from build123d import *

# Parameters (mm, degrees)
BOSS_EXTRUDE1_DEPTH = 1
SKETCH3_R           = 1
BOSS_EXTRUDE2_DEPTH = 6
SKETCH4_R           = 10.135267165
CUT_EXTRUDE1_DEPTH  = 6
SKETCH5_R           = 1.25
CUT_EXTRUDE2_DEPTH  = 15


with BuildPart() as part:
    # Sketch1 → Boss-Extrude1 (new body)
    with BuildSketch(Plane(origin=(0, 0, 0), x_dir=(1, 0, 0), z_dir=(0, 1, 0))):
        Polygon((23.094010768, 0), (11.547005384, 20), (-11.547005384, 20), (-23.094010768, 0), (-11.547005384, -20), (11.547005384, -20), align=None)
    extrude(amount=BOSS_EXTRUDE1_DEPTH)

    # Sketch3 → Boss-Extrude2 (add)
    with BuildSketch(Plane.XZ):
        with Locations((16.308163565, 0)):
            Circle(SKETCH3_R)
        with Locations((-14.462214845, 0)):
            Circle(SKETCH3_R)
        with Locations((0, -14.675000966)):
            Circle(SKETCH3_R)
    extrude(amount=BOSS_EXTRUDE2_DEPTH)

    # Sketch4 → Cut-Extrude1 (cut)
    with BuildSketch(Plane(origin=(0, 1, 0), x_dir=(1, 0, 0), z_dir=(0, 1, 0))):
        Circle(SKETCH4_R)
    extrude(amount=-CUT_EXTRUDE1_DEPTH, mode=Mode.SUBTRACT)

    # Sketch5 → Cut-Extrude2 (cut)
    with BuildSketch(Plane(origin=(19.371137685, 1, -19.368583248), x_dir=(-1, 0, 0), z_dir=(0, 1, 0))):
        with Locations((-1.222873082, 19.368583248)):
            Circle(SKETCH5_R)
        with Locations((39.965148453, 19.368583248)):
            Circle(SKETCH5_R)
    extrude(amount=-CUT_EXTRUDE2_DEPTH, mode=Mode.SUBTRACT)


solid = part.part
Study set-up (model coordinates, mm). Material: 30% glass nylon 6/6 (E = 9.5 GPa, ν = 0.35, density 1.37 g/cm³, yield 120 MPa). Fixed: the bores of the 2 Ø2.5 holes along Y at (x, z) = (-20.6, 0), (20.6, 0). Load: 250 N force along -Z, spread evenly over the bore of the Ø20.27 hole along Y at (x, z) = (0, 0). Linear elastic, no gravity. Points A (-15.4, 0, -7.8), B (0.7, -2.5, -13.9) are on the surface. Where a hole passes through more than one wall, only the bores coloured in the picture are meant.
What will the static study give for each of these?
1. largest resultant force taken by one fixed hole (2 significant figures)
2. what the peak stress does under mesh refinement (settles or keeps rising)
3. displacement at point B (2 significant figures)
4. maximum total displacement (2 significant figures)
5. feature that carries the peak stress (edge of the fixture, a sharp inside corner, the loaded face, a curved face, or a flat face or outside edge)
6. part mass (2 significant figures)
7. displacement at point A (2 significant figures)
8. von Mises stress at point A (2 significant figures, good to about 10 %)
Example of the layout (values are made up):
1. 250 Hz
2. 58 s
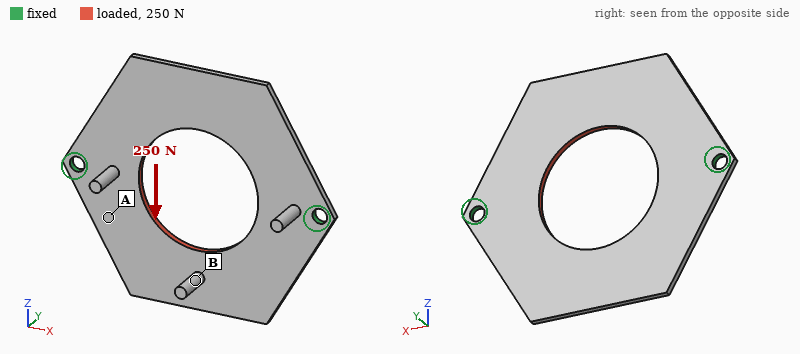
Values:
1. 130 N
2. keeps rising
3. 31 µm
4. 33 µm
5. edge of the fixture
6. 1.5 g
7. 20 µm
8. 9.7 MPa
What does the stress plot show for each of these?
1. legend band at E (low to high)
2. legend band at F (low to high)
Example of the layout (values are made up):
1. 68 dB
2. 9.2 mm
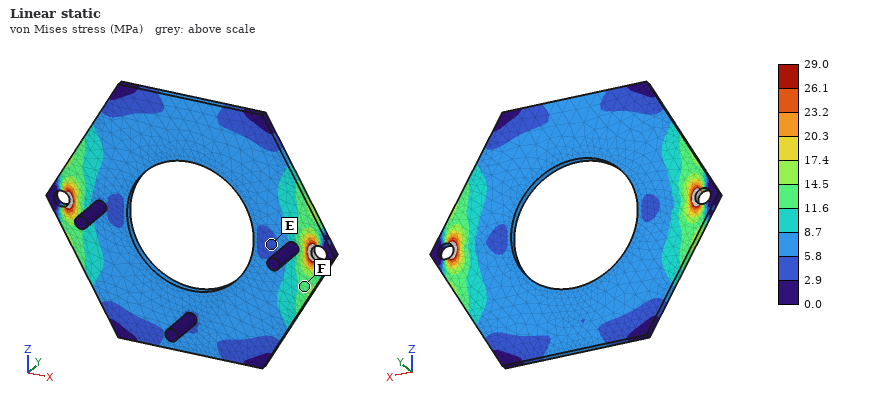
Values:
1. 2.9 to 5.8 MPa
2. 11.6 to 14.5 MPa
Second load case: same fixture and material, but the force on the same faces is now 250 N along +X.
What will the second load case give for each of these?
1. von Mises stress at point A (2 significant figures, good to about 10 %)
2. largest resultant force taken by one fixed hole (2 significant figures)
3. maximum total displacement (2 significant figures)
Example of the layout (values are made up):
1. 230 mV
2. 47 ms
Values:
1. 5.8 MPa
2. 130 N
3. 27 µm
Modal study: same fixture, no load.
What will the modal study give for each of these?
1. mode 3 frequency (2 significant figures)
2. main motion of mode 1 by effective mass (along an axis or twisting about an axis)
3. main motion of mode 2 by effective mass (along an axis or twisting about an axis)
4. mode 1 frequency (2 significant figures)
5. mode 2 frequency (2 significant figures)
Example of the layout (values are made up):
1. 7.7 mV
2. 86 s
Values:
1. 2000 Hz
2. twisting about X
3. along Y
4. 650 Hz
5. 820 Hz
